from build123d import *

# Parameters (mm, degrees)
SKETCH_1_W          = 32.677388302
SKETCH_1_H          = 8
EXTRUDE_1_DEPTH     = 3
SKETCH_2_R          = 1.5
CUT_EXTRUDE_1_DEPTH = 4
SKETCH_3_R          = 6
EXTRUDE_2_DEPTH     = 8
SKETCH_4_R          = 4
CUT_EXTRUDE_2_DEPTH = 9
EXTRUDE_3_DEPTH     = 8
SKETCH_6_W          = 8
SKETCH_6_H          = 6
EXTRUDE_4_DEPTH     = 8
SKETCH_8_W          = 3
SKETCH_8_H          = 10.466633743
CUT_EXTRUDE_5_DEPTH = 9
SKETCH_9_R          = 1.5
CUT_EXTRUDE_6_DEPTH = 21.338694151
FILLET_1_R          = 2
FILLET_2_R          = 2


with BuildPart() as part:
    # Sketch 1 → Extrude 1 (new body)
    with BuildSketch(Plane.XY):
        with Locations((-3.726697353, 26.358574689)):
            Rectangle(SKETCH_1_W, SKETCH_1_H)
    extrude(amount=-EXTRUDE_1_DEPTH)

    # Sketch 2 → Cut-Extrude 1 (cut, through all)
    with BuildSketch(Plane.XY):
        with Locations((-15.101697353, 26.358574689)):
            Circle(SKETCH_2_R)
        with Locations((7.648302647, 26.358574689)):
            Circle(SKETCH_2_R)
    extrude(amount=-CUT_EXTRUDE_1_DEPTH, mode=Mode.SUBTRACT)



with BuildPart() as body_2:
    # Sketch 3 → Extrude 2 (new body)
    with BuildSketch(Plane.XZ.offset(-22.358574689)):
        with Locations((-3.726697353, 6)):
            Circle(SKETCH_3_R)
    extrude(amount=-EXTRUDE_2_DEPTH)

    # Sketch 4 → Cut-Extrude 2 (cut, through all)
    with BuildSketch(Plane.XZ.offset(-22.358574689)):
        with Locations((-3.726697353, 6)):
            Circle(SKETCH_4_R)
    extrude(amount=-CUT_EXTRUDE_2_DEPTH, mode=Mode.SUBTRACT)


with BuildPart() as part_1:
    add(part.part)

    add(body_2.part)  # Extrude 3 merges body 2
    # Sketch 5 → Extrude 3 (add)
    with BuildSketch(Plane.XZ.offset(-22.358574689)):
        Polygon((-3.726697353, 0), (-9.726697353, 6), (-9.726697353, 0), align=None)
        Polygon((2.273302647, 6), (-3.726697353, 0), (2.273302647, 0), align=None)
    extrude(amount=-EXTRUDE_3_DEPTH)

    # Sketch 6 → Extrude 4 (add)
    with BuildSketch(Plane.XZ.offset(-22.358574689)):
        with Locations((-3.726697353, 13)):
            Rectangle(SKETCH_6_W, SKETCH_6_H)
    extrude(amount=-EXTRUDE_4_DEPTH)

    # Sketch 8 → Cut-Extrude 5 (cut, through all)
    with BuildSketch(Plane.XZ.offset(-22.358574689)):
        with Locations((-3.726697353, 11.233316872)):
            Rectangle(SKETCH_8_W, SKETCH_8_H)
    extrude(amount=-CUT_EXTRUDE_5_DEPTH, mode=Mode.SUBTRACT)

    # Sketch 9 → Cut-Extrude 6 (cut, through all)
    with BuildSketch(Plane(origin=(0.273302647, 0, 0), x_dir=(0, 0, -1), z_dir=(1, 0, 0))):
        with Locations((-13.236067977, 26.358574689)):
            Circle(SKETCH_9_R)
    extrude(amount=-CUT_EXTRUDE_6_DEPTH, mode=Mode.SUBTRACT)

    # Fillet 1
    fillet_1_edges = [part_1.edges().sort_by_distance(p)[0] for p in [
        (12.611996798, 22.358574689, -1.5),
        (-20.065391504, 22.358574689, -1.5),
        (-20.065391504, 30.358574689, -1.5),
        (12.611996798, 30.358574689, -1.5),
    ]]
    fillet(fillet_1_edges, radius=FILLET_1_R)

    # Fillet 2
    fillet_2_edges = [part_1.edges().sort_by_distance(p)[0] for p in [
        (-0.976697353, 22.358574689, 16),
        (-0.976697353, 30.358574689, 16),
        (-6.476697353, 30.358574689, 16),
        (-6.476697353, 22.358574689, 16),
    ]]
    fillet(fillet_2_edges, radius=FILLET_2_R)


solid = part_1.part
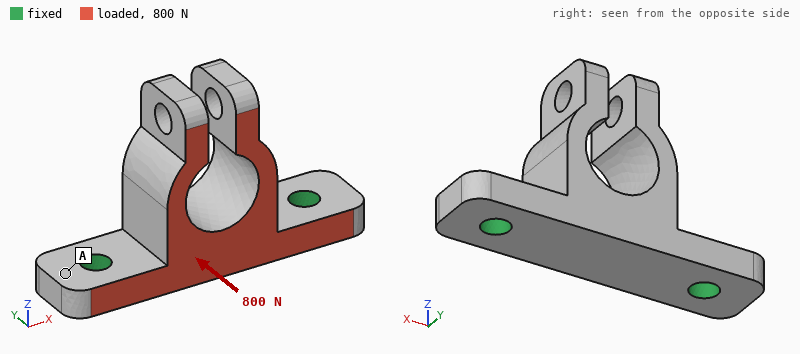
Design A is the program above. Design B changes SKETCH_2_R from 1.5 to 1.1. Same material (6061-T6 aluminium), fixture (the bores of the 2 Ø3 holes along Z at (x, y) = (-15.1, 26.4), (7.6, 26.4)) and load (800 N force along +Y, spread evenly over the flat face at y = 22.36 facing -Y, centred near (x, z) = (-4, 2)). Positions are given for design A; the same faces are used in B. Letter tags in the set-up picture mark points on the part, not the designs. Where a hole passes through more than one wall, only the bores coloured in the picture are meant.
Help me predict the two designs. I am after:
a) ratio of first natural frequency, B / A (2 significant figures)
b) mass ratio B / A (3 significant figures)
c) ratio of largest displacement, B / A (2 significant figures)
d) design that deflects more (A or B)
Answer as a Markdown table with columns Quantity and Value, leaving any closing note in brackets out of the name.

| Quantity | Value |
|---|---|
| ratio of first natural frequency, B / A | 0.93 |
| mass ratio B / A | 1.01 |
| ratio of largest displacement, B / A | 1.1 |
| design that deflects more | B |
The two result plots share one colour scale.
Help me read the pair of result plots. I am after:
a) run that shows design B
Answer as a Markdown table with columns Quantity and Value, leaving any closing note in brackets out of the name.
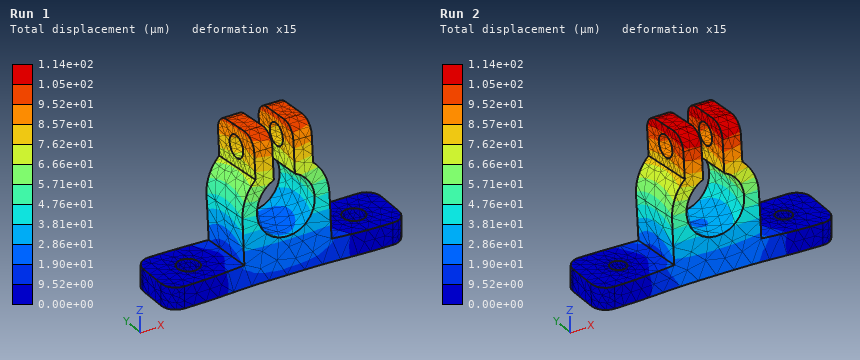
| Quantity | Value |
|---|---|
| run that shows design B | Run 2 |
